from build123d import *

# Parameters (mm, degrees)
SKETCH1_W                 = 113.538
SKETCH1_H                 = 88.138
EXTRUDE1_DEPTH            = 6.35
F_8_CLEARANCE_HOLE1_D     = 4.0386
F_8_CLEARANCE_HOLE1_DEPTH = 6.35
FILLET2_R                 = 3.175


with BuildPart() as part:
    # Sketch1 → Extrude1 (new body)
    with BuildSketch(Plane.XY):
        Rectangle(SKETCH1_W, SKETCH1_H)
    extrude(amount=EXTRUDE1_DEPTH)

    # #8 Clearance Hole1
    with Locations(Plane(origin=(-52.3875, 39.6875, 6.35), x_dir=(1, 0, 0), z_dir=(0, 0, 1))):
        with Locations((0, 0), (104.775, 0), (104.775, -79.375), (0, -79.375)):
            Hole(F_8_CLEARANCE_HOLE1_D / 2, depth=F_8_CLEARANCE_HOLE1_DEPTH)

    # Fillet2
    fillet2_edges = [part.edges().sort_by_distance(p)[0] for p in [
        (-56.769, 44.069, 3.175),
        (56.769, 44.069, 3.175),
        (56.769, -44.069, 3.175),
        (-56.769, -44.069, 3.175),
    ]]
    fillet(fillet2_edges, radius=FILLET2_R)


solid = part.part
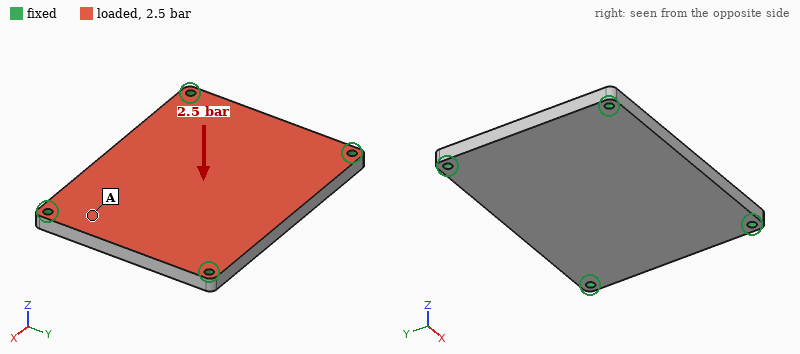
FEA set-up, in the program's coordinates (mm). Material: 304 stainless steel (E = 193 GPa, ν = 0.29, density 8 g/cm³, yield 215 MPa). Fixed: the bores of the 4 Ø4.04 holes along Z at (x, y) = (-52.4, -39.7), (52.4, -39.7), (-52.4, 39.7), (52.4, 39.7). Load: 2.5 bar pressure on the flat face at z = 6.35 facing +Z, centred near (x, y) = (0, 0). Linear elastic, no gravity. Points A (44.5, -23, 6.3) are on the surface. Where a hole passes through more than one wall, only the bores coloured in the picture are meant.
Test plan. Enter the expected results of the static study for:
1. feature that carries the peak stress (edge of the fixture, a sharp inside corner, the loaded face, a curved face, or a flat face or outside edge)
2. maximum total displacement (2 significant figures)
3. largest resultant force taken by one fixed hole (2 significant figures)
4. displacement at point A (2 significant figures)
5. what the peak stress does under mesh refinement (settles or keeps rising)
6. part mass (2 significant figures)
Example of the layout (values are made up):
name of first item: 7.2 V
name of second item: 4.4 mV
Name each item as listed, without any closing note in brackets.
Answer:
feature that carries the peak stress: edge of the fixture
maximum total displacement: 42 µm
largest resultant force taken by one fixed hole: 620 N
displacement at point A: 12 µm
what the peak stress does under mesh refinement: keeps rising
part mass: 510 g
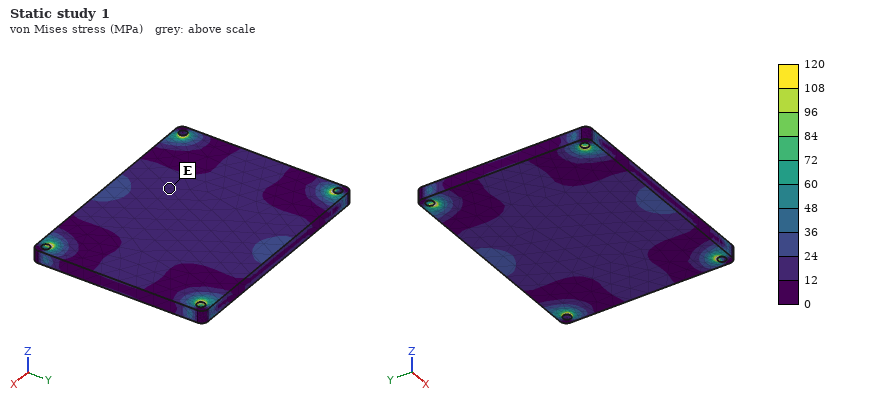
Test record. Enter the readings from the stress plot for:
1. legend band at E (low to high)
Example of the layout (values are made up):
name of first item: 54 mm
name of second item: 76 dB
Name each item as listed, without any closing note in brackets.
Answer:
legend band at E: 12 to 24 MPa
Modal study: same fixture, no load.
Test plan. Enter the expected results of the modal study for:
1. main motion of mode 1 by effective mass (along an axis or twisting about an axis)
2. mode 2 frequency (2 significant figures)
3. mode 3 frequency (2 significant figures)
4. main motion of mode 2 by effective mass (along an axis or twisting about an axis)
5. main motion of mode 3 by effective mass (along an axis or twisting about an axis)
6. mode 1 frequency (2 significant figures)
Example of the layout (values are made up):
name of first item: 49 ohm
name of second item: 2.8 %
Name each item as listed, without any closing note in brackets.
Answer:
main motion of mode 1 by effective mass: along Z
mode 2 frequency: 3400 Hz
mode 3 frequency: 4400 Hz
main motion of mode 2 by effective mass: twisting about X
main motion of mode 3 by effective mass: twisting about Y
mode 1 frequency: 2000 Hz
